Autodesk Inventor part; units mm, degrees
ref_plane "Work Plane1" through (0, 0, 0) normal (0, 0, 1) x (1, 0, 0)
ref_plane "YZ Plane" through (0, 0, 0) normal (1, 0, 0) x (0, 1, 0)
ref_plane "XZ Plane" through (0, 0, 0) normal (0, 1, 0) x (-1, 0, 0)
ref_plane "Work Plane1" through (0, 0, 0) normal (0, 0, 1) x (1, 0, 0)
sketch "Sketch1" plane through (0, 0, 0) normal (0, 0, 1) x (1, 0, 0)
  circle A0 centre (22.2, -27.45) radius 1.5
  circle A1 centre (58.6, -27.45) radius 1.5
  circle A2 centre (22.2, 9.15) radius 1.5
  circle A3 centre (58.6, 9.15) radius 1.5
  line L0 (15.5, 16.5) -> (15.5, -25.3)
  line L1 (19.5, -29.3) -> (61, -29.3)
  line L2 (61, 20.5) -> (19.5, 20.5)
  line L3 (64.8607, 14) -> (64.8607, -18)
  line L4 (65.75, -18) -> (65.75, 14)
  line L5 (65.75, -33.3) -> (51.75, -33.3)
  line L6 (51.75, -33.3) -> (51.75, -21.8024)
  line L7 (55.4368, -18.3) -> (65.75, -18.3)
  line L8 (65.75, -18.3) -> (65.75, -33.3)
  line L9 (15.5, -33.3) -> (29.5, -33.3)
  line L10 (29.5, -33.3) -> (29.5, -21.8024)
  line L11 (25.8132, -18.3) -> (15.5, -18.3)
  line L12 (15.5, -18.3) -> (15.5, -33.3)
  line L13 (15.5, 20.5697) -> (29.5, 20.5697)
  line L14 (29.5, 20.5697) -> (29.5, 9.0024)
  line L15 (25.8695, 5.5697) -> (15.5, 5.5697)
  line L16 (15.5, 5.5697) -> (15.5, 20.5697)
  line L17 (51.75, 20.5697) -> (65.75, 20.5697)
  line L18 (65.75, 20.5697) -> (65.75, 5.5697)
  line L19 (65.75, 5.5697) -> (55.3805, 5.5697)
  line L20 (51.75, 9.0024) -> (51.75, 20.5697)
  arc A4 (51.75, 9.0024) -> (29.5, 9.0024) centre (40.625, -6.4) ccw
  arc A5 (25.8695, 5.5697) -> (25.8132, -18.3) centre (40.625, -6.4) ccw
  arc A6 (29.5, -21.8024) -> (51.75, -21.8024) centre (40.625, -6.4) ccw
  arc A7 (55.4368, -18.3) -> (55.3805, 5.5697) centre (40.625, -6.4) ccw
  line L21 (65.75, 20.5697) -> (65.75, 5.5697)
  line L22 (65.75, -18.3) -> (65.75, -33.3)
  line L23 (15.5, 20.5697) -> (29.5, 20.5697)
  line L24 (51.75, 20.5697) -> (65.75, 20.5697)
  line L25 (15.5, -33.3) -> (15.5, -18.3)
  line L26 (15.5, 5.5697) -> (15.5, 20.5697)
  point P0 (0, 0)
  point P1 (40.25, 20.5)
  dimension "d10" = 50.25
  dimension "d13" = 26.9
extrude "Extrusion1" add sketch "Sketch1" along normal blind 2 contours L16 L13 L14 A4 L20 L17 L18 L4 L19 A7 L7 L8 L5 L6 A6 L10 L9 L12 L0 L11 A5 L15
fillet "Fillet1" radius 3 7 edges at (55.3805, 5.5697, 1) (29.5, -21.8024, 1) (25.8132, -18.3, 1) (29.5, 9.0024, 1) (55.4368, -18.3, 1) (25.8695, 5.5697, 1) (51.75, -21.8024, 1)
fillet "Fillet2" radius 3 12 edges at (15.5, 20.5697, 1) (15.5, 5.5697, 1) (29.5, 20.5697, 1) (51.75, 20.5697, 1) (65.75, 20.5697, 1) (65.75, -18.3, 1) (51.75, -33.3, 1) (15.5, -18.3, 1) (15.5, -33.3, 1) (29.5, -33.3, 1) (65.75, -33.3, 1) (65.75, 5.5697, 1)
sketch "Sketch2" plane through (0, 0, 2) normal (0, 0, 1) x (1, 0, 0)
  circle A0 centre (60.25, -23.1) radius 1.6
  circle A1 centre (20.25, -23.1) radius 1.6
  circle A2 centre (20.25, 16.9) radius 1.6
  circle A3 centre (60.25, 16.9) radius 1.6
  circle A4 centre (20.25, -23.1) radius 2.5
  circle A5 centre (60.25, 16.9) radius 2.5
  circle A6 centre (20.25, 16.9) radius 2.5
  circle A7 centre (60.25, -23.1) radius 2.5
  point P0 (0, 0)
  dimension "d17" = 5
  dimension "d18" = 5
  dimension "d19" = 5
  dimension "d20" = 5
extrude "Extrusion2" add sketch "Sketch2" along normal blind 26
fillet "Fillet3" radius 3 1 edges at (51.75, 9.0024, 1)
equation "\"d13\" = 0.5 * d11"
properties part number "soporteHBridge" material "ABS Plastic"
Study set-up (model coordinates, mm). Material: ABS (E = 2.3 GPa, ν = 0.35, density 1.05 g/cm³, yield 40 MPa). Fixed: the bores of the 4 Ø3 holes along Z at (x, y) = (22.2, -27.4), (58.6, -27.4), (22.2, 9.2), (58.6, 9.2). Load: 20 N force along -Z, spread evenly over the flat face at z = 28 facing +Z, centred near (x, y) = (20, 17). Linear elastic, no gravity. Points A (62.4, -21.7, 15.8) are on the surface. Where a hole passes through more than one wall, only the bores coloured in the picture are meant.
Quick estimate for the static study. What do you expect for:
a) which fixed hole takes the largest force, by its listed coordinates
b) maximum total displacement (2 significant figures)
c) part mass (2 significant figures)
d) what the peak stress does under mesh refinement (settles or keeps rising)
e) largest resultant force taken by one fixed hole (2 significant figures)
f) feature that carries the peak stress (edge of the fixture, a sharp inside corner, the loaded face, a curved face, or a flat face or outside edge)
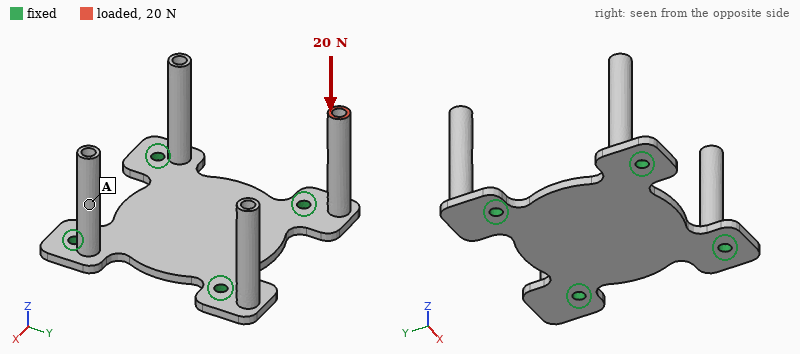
(22.2, 9.2)
0.78 mm
5.3 g
keeps rising
21 N
edge of the fixture
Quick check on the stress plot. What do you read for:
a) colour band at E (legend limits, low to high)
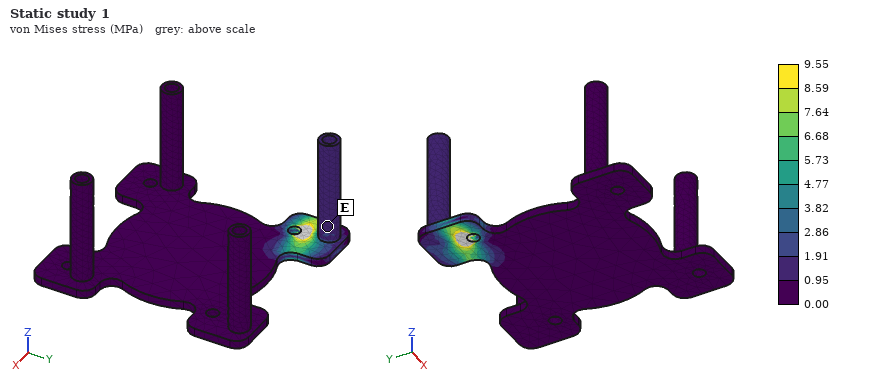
0.95 to 1.91 MPa
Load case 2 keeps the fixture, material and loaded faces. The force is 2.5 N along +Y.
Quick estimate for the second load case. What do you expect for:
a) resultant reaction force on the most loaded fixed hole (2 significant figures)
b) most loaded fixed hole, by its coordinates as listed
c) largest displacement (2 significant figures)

2.7 N
(22.2, 9.2)
0.88 mm
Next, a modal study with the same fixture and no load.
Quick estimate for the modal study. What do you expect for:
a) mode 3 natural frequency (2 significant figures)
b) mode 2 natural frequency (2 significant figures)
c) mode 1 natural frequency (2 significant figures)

990 Hz
830 Hz
820 Hz
